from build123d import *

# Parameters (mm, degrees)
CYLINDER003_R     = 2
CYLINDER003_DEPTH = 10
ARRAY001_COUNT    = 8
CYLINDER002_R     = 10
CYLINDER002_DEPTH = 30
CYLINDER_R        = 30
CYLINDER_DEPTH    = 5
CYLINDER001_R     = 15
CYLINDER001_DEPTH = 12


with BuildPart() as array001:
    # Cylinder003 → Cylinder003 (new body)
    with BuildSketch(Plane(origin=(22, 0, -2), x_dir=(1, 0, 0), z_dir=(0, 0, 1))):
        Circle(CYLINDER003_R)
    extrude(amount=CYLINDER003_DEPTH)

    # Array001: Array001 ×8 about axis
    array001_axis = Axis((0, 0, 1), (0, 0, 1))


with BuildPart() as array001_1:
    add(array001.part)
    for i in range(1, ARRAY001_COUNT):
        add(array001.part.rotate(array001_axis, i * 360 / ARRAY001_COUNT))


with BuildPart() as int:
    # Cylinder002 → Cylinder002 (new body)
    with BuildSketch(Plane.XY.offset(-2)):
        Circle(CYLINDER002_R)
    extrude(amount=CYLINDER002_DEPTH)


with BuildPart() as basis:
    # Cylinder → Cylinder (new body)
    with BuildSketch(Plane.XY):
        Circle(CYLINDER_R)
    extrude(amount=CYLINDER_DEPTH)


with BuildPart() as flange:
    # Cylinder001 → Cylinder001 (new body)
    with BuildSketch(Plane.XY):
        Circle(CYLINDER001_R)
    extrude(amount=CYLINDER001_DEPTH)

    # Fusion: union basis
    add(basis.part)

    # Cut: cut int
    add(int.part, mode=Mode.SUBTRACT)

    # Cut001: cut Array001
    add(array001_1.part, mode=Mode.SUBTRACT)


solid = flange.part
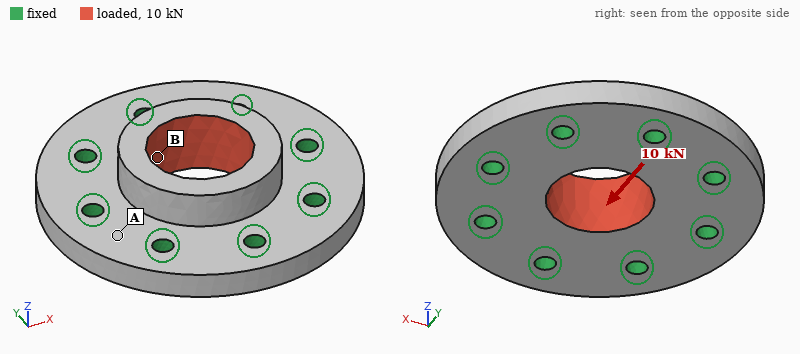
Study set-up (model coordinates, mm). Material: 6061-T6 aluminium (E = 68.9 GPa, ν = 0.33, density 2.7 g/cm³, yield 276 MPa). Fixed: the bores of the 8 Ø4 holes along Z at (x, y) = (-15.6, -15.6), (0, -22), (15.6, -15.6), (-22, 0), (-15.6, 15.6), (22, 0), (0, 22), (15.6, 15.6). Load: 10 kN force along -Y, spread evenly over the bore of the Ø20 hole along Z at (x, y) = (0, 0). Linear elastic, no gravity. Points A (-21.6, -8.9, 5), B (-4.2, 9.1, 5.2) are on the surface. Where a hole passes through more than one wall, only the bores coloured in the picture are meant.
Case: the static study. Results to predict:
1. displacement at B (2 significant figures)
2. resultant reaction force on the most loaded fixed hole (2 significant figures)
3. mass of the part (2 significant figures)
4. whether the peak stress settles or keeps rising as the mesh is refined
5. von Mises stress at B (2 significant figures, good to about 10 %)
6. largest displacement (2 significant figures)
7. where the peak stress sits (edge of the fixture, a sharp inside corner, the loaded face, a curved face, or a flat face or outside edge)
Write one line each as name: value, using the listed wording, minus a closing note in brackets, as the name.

displacement at B: 6.3 µm
resultant reaction force on the most loaded fixed hole: 1.9 kN
mass of the part: 40 g
whether the peak stress settles or keeps rising as the mesh is refined: keeps rising
von Mises stress at B: 29 MPa
largest displacement: 14 µm
where the peak stress sits: edge of the fixture
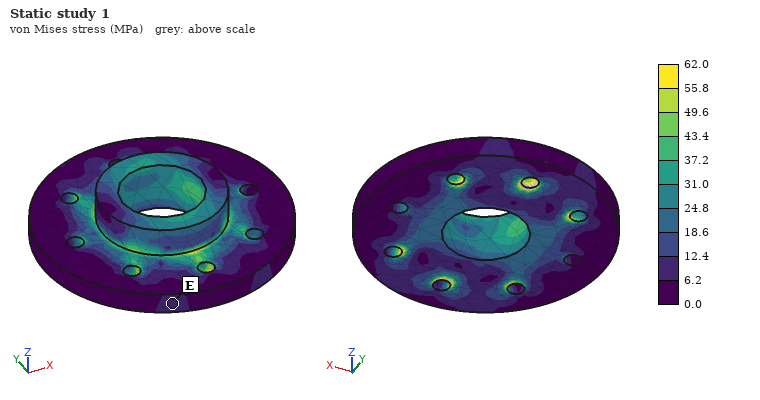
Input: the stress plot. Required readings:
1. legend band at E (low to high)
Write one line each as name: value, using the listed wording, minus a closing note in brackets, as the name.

legend band at E: 6.2 to 12.4 MPa
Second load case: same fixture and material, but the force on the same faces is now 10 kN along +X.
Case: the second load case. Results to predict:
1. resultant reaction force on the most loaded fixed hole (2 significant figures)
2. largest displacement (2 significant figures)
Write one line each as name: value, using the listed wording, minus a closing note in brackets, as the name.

resultant reaction force on the most loaded fixed hole: 1.9 kN
largest displacement: 14 µm
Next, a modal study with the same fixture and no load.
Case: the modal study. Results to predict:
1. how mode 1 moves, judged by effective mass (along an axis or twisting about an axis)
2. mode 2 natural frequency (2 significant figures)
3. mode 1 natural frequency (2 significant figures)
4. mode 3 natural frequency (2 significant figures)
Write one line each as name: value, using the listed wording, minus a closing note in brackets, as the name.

how mode 1 moves, judged by effective mass: along Z
mode 2 natural frequency: 38 kHz
mode 1 natural frequency: 30 kHz
mode 3 natural frequency: 38 kHz
